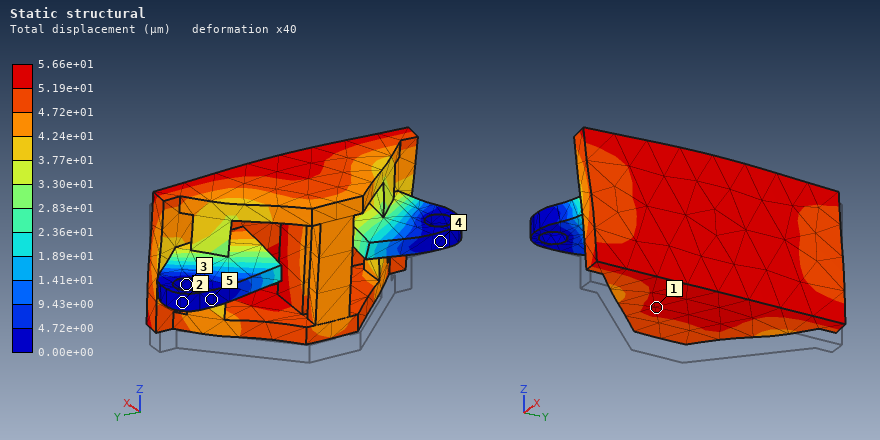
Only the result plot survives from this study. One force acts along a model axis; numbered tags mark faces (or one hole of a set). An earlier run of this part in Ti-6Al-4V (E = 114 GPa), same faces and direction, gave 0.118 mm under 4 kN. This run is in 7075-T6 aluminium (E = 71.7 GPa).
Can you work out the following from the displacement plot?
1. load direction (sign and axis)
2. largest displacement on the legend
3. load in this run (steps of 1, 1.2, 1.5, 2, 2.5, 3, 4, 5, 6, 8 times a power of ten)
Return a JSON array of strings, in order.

["+Z", "5.66e+01 µm", "1.2 kN"]
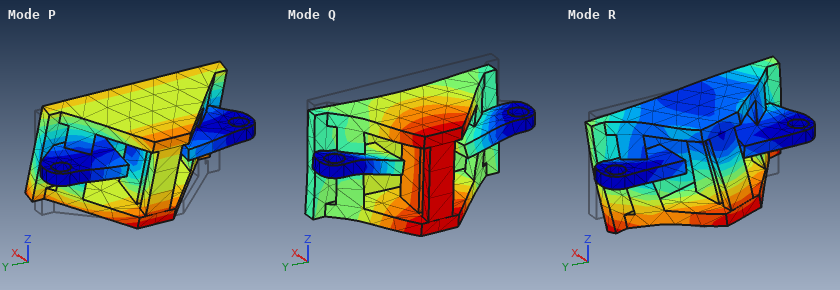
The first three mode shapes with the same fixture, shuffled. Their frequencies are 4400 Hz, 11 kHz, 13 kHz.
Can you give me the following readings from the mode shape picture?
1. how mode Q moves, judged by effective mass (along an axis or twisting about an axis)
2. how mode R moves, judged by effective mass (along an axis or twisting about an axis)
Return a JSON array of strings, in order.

["along Z", "along Y"]
